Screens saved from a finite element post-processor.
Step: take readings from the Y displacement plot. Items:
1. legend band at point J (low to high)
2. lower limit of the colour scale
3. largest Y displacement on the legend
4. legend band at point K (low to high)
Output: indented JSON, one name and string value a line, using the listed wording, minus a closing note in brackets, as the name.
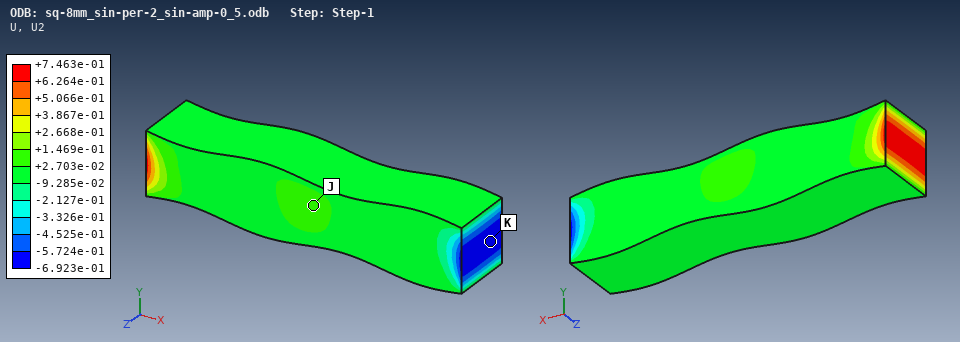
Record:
{
  "legend band at point J": "+2.703e-02 to +1.469e-01",
  "lower limit of the colour scale": "-6.923e-01",
  "largest Y displacement on the legend": "+7.463e-01",
  "legend band at point K": "-6.923e-01 to -5.724e-01"
}
